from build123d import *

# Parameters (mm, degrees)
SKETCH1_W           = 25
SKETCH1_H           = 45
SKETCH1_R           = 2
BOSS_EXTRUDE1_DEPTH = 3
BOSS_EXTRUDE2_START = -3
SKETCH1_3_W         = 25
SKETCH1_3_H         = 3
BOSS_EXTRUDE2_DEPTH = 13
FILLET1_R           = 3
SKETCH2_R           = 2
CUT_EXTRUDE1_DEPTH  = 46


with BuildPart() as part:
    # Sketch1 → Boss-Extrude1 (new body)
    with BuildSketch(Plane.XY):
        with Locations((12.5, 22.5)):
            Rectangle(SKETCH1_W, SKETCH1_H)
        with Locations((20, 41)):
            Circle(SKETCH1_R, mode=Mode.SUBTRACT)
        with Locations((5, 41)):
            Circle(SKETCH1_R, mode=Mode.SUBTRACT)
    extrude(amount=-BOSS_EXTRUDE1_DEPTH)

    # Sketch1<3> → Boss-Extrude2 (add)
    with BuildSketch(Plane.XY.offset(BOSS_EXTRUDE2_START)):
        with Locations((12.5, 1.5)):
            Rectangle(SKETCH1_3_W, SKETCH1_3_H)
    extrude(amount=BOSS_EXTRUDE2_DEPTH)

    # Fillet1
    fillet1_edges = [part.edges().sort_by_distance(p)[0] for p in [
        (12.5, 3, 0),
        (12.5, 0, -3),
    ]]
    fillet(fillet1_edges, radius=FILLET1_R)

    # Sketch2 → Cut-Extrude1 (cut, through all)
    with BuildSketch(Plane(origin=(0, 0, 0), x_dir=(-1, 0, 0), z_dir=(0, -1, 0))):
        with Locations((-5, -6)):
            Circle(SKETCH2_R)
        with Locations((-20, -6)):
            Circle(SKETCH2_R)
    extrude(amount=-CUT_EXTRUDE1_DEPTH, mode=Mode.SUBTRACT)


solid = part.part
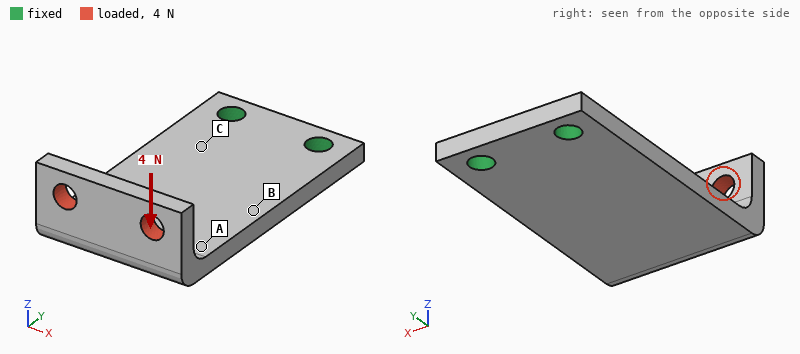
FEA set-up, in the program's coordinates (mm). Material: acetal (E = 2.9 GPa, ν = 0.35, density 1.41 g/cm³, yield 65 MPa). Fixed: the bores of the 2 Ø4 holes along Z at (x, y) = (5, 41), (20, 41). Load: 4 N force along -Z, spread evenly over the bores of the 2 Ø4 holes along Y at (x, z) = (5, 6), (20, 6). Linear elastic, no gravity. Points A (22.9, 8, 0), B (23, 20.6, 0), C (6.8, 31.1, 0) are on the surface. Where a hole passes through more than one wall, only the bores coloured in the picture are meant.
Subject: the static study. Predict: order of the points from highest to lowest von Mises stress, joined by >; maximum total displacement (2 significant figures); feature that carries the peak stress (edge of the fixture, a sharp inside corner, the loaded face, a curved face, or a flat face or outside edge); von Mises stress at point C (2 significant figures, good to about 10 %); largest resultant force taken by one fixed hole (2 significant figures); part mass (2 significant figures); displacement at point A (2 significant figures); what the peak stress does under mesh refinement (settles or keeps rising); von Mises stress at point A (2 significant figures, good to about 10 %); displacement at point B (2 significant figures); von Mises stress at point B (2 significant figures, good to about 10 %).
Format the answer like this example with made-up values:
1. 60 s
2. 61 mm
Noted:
1. C > B > A
2. 0.52 mm
3. edge of the fixture
4. 2.9 MPa
5. 2.0 N
6. 5.6 g
7. 0.34 mm
8. keeps rising
9. 0.73 MPa
10. 0.14 mm
11. 2.1 MPa
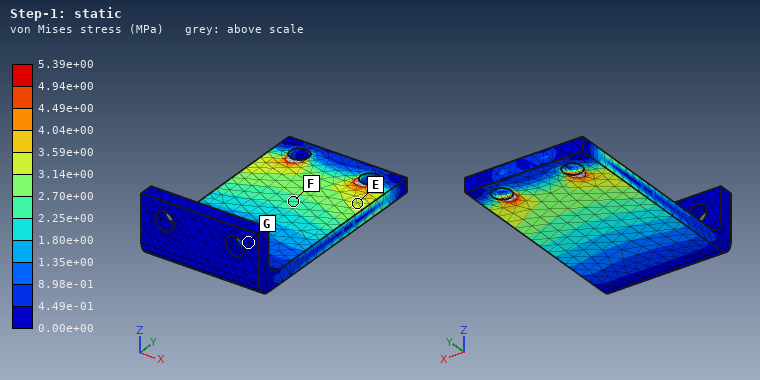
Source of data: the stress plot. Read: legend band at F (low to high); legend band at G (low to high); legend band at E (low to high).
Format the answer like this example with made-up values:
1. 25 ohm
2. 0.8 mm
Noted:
1. 2.25e+00 to 2.70e+00 MPa
2. 0.00e+00 to 4.49e-01 MPa
3. 3.14e+00 to 3.59e+00 MPa
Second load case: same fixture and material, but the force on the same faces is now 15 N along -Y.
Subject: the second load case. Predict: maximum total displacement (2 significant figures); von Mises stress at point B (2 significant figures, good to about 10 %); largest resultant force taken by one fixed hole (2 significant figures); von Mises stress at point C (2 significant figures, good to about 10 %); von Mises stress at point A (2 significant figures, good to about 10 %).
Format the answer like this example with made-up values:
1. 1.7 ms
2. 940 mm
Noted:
1. 0.61 mm
2. 3.2 MPa
3. 7.6 N
4. 3.0 MPa
5. 3.0 MPa
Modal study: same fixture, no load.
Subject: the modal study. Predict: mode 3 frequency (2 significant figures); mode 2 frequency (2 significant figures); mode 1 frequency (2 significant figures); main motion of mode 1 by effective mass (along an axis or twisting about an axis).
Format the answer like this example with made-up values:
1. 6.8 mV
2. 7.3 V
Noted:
1. 1900 Hz
2. 1000 Hz
3. 320 Hz
4. along Z
